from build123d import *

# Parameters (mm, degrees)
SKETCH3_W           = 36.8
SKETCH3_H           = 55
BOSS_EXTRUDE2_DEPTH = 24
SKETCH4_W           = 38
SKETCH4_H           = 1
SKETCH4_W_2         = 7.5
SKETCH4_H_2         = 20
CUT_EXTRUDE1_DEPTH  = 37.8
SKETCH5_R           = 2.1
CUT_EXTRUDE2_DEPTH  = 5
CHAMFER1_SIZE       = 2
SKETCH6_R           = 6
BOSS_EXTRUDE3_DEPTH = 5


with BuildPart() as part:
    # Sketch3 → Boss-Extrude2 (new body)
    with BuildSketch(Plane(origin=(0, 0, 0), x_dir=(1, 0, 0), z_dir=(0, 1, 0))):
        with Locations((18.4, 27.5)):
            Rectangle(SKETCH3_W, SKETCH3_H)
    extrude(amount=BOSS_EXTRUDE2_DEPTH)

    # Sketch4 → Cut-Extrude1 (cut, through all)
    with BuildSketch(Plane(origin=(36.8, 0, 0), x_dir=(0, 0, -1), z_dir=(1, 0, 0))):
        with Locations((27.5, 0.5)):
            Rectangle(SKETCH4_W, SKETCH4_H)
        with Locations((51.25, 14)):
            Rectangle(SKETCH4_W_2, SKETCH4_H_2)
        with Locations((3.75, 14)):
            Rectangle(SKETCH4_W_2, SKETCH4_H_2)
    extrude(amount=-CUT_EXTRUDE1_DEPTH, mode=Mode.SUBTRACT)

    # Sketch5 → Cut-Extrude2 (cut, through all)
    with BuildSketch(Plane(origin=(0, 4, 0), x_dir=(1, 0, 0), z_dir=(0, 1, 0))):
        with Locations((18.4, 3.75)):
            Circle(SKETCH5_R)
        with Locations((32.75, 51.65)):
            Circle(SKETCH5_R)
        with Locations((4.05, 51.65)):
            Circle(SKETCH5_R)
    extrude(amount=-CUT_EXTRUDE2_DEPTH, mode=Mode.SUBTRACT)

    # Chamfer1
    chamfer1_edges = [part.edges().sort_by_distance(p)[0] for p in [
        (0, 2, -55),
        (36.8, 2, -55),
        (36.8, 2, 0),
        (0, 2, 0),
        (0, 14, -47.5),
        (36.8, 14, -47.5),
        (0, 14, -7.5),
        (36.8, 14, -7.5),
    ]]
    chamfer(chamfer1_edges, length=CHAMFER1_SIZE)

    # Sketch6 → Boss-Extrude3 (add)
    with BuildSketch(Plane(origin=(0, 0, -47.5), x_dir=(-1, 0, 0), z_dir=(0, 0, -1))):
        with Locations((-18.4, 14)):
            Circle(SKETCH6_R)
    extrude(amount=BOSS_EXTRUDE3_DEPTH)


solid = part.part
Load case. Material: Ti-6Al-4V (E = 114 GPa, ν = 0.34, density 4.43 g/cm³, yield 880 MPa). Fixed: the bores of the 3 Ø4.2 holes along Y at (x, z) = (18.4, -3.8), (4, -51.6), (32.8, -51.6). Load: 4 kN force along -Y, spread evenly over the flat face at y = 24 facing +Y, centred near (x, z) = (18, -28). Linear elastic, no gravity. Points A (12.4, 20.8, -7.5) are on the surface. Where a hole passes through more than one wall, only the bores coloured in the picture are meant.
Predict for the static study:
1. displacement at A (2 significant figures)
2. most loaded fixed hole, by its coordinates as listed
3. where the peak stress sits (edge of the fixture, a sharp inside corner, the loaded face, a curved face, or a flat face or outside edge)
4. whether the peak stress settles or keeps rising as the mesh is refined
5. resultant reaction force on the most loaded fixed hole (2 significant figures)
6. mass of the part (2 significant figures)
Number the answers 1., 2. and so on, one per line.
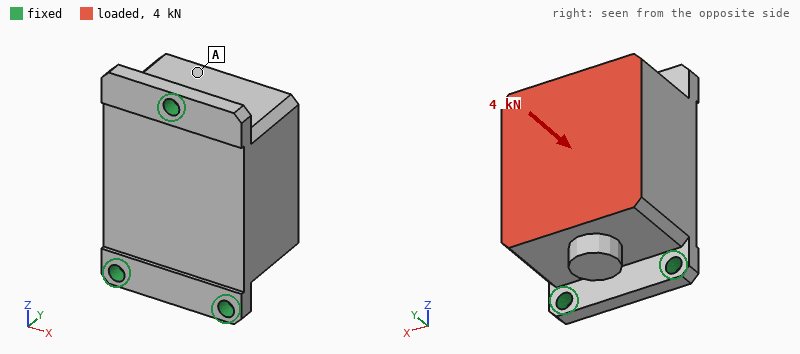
1. 8.5 µm
2. (18.4, -3.8)
3. edge of the fixture
4. keeps rising
5. 2.3 kN
6. 160 g
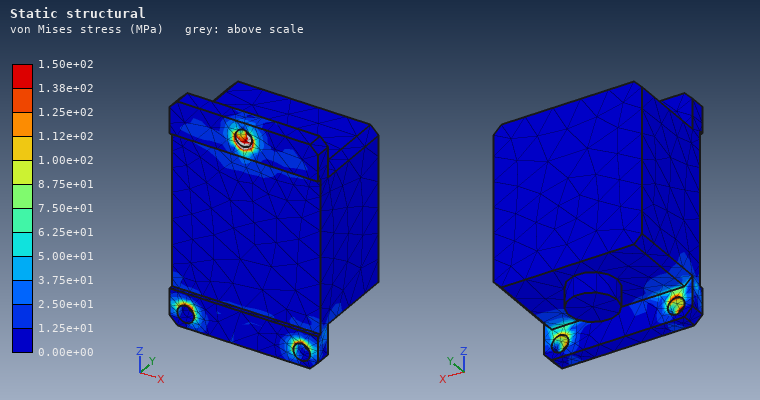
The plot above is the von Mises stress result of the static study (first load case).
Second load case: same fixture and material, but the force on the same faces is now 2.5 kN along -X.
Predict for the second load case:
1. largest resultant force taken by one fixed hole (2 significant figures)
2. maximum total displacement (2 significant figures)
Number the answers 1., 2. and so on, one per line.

1. 2.4 kN
2. 28 µm
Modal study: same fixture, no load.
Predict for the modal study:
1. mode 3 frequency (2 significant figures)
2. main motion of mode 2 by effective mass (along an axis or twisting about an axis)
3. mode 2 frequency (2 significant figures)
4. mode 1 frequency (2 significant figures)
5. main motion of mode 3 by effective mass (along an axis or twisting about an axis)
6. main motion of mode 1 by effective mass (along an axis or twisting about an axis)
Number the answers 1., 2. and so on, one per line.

1. 12 kHz
2. along Y
3. 9200 Hz
4. 6100 Hz
5. along Z
6. along X
